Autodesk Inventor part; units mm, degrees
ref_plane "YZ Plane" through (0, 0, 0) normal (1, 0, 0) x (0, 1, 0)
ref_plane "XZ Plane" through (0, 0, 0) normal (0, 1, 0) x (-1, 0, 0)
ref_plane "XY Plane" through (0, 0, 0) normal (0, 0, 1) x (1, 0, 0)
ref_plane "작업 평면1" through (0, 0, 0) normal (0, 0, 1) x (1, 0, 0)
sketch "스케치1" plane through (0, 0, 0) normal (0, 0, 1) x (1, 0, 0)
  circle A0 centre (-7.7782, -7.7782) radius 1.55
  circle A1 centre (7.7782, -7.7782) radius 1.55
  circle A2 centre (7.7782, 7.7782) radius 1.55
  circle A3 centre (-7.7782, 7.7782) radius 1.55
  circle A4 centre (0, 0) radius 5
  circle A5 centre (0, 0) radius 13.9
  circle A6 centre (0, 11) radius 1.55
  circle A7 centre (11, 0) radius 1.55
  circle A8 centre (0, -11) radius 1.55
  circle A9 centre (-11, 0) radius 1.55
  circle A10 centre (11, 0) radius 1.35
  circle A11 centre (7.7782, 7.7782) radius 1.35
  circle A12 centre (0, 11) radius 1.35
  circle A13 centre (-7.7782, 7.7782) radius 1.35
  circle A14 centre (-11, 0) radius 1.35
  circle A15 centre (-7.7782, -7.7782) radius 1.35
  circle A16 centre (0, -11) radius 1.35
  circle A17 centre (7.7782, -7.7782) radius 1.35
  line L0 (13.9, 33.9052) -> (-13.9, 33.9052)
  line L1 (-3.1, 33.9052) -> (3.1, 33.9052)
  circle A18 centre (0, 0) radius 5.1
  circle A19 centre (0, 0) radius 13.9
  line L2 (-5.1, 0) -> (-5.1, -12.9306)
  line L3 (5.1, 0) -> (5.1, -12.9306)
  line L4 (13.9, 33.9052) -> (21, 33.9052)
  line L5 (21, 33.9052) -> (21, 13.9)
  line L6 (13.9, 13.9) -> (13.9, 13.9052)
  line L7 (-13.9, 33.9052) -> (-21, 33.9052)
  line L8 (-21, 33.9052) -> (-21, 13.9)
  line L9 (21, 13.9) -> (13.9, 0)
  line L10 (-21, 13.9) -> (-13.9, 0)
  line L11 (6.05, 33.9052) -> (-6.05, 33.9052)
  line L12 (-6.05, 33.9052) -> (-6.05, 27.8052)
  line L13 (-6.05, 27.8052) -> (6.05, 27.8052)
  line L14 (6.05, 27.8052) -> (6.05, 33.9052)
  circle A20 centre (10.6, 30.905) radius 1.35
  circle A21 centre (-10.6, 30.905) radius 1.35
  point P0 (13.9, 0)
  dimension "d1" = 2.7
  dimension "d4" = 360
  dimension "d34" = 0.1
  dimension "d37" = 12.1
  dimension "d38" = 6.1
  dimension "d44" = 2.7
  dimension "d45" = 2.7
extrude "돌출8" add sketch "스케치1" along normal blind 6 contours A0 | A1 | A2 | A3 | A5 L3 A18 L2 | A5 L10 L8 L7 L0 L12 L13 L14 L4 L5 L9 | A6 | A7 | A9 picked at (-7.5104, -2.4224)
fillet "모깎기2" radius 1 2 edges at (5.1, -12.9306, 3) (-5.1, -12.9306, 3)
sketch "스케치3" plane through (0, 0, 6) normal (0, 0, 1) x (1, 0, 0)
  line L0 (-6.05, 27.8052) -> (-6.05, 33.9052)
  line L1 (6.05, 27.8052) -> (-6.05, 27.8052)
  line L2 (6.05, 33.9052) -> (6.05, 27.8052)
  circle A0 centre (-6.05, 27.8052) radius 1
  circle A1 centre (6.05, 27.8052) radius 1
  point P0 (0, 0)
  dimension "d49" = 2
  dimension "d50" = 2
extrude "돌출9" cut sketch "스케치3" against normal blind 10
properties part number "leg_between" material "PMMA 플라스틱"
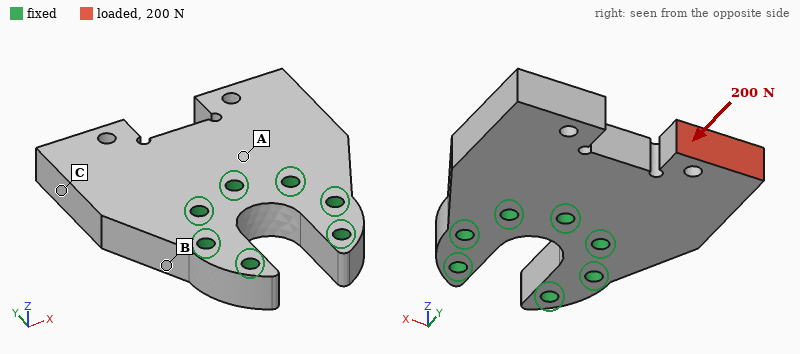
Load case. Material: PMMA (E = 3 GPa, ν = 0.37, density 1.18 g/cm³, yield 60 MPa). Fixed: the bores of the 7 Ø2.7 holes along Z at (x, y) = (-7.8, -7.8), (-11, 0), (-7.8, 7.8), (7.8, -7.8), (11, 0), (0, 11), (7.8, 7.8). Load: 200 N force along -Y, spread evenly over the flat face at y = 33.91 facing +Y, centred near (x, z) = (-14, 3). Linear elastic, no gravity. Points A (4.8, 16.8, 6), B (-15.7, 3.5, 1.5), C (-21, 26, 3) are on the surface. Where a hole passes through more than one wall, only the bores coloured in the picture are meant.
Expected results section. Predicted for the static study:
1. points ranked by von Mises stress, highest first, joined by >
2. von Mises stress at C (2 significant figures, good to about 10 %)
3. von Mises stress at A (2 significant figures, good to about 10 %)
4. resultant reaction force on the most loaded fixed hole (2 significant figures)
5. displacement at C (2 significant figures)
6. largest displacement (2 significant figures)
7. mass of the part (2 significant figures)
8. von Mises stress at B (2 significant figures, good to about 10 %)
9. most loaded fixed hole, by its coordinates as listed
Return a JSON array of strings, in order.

["B > C > A", "2.3 MPa", "0.76 MPa", "120 N", "33 µm", "42 µm", "9.3 g", "3.3 MPa", "(-7.8, 7.8)"]
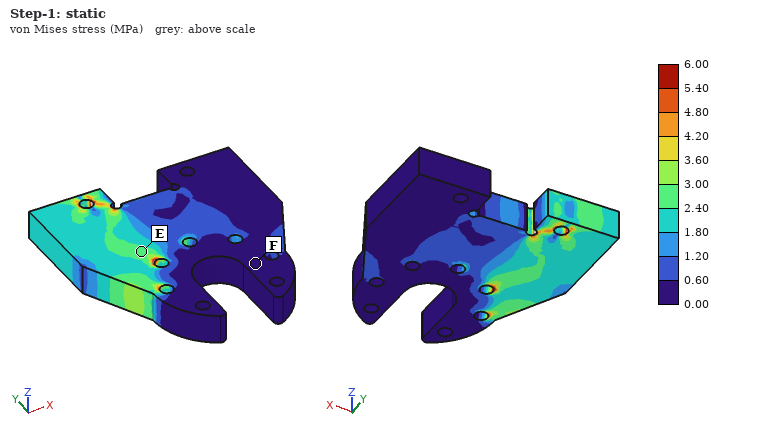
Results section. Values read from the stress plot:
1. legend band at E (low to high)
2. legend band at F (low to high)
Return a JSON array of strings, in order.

["2.40 to 3.00 MPa", "0.00 to 0.60 MPa"]
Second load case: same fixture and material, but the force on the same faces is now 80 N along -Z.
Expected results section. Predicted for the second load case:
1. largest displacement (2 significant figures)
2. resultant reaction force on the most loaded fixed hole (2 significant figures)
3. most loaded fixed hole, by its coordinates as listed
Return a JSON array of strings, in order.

["0.45 mm", "83 N", "(0, 11)"]
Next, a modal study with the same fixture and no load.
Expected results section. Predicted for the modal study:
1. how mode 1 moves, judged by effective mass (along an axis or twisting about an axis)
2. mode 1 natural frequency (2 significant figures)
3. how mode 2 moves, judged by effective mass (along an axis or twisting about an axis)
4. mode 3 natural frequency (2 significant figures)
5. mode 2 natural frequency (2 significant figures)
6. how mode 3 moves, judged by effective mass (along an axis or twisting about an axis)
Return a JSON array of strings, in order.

["along Z", "2500 Hz", "twisting about Y", "5800 Hz", "2700 Hz", "along X"]
